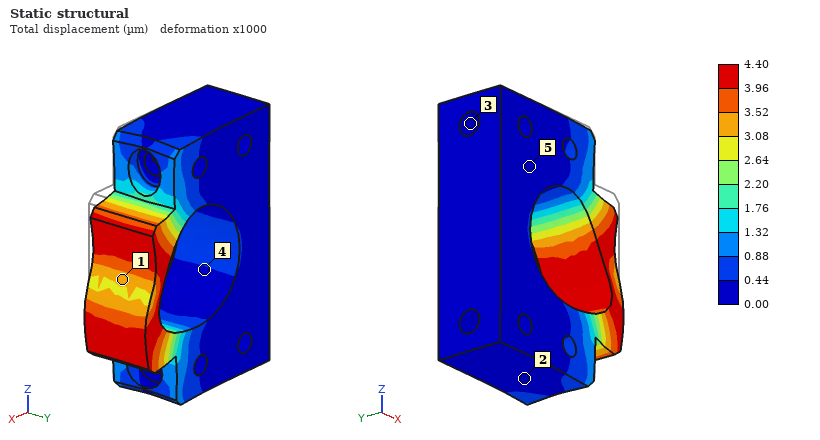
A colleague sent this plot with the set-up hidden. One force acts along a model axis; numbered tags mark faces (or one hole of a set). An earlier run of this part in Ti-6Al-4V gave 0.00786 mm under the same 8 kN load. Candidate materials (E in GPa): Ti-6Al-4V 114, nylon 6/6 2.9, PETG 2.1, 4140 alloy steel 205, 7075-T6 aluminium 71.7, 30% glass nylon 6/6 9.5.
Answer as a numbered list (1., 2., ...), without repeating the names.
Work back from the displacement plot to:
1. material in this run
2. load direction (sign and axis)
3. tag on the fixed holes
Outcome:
1. 4140 alloy steel
2. -Z
3. 3
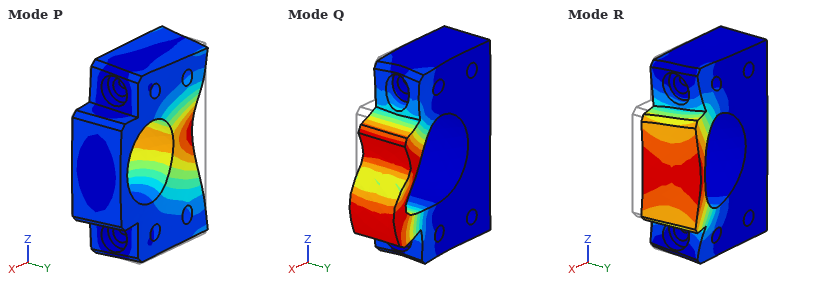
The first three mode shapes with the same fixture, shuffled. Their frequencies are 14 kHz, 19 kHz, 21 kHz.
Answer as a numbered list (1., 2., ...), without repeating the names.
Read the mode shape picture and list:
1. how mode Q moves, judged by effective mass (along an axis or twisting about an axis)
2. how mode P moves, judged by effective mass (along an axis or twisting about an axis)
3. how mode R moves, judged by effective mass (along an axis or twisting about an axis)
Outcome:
1. along Z
2. along Y
3. along Y
